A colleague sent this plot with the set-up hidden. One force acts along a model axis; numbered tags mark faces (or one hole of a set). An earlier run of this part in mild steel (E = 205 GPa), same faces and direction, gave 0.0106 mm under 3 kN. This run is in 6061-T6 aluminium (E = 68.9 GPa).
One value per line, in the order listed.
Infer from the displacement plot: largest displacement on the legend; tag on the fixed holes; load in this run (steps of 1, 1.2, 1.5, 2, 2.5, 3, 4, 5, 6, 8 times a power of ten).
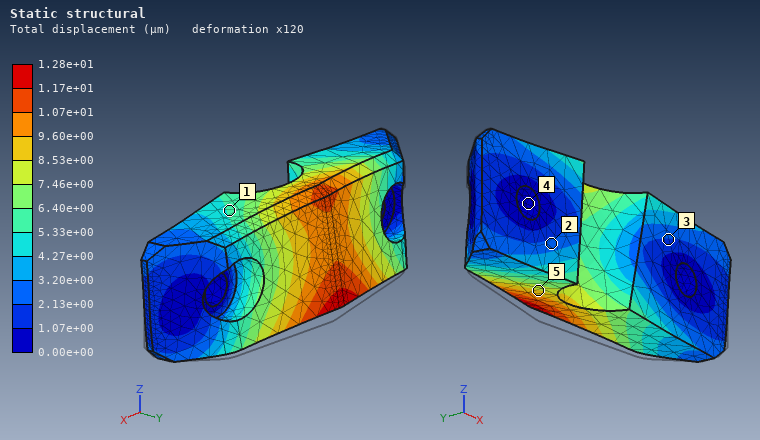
1.28e+01 µm
4
1.2 kN
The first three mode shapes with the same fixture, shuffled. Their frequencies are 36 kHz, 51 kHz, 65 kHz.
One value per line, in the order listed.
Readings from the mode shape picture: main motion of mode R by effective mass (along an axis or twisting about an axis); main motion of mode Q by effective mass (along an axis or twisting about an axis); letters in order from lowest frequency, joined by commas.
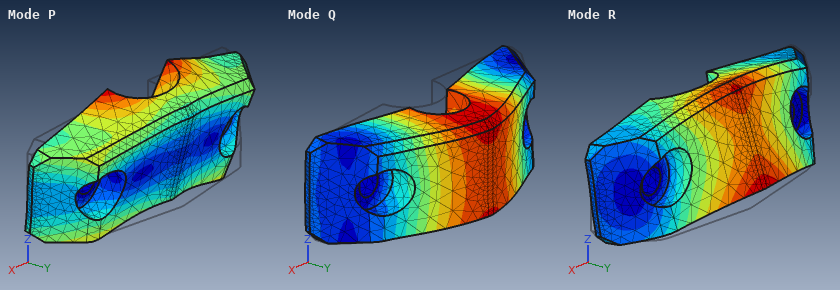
along Z
along Y
R, Q, P
